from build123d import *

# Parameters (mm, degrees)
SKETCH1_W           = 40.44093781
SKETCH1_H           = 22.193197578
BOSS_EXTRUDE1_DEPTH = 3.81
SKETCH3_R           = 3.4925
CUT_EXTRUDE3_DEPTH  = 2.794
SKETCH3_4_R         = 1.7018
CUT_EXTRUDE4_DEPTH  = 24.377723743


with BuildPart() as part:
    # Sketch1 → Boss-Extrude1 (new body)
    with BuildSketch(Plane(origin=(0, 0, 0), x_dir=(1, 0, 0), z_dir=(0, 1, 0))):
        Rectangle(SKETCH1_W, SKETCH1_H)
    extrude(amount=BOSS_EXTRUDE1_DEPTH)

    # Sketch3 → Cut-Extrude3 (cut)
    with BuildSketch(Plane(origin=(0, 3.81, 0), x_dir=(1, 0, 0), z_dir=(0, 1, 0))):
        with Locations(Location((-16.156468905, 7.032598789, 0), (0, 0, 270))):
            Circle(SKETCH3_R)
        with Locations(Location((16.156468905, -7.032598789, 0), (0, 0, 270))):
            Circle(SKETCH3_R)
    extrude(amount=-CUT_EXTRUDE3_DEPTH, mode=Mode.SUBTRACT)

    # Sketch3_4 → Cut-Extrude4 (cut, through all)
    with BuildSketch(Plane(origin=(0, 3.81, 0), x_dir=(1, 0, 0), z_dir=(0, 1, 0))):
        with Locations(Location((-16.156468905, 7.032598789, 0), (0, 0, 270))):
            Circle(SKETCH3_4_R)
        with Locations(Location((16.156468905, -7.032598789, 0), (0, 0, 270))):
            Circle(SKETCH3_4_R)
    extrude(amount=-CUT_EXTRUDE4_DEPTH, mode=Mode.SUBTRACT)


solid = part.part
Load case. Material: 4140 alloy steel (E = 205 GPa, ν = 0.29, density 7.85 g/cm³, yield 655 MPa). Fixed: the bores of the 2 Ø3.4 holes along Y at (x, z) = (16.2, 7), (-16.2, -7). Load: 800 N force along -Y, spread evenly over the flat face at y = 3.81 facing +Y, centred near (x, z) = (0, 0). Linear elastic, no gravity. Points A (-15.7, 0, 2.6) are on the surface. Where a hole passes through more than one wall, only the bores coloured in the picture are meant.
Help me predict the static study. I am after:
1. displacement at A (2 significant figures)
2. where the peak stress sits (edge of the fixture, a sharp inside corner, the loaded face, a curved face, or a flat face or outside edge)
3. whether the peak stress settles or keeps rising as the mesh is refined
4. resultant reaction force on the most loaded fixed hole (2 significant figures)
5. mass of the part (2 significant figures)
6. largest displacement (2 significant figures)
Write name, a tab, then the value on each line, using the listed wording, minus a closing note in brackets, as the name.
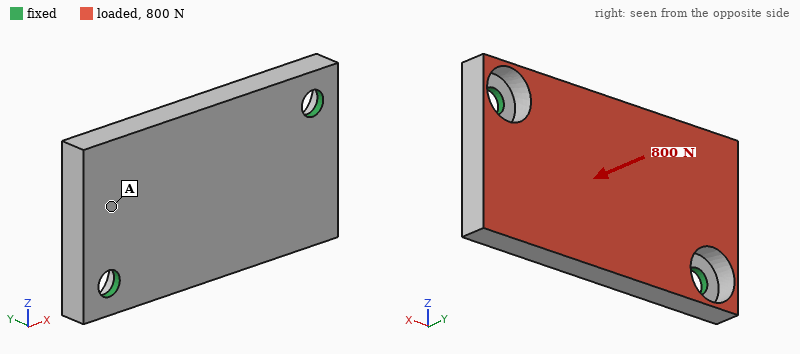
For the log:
displacement at A	11 µm
where the peak stress sits	edge of the fixture
whether the peak stress settles or keeps rising as the mesh is refined	keeps rising
resultant reaction force on the most loaded fixed hole	670 N
mass of the part	25 g
largest displacement	20 µm
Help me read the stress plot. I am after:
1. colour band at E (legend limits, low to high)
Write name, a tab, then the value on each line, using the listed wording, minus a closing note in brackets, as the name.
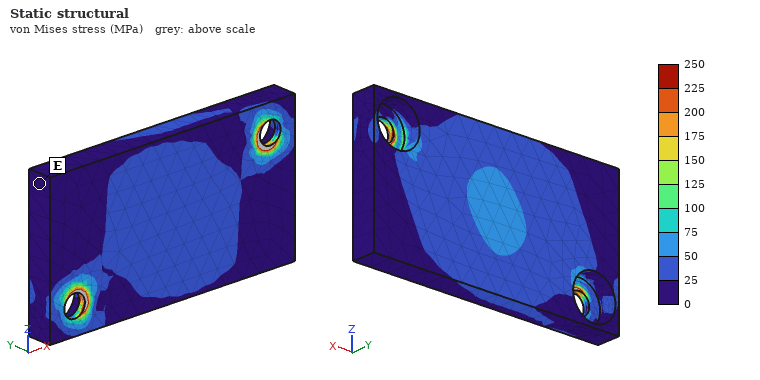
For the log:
colour band at E	0 to 25 MPa
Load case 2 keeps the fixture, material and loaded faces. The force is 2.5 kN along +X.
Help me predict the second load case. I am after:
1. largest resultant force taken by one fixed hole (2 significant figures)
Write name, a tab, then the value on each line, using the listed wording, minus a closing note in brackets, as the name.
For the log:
largest resultant force taken by one fixed hole	1.3 kN
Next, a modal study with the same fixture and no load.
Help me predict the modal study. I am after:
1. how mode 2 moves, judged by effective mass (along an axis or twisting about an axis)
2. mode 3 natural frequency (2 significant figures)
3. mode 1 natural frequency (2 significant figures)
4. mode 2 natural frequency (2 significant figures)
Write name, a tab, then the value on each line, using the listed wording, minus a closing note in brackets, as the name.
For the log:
how mode 2 moves, judged by effective mass	along Y
mode 3 natural frequency	14 kHz
mode 1 natural frequency	4100 Hz
mode 2 natural frequency	7800 Hz
